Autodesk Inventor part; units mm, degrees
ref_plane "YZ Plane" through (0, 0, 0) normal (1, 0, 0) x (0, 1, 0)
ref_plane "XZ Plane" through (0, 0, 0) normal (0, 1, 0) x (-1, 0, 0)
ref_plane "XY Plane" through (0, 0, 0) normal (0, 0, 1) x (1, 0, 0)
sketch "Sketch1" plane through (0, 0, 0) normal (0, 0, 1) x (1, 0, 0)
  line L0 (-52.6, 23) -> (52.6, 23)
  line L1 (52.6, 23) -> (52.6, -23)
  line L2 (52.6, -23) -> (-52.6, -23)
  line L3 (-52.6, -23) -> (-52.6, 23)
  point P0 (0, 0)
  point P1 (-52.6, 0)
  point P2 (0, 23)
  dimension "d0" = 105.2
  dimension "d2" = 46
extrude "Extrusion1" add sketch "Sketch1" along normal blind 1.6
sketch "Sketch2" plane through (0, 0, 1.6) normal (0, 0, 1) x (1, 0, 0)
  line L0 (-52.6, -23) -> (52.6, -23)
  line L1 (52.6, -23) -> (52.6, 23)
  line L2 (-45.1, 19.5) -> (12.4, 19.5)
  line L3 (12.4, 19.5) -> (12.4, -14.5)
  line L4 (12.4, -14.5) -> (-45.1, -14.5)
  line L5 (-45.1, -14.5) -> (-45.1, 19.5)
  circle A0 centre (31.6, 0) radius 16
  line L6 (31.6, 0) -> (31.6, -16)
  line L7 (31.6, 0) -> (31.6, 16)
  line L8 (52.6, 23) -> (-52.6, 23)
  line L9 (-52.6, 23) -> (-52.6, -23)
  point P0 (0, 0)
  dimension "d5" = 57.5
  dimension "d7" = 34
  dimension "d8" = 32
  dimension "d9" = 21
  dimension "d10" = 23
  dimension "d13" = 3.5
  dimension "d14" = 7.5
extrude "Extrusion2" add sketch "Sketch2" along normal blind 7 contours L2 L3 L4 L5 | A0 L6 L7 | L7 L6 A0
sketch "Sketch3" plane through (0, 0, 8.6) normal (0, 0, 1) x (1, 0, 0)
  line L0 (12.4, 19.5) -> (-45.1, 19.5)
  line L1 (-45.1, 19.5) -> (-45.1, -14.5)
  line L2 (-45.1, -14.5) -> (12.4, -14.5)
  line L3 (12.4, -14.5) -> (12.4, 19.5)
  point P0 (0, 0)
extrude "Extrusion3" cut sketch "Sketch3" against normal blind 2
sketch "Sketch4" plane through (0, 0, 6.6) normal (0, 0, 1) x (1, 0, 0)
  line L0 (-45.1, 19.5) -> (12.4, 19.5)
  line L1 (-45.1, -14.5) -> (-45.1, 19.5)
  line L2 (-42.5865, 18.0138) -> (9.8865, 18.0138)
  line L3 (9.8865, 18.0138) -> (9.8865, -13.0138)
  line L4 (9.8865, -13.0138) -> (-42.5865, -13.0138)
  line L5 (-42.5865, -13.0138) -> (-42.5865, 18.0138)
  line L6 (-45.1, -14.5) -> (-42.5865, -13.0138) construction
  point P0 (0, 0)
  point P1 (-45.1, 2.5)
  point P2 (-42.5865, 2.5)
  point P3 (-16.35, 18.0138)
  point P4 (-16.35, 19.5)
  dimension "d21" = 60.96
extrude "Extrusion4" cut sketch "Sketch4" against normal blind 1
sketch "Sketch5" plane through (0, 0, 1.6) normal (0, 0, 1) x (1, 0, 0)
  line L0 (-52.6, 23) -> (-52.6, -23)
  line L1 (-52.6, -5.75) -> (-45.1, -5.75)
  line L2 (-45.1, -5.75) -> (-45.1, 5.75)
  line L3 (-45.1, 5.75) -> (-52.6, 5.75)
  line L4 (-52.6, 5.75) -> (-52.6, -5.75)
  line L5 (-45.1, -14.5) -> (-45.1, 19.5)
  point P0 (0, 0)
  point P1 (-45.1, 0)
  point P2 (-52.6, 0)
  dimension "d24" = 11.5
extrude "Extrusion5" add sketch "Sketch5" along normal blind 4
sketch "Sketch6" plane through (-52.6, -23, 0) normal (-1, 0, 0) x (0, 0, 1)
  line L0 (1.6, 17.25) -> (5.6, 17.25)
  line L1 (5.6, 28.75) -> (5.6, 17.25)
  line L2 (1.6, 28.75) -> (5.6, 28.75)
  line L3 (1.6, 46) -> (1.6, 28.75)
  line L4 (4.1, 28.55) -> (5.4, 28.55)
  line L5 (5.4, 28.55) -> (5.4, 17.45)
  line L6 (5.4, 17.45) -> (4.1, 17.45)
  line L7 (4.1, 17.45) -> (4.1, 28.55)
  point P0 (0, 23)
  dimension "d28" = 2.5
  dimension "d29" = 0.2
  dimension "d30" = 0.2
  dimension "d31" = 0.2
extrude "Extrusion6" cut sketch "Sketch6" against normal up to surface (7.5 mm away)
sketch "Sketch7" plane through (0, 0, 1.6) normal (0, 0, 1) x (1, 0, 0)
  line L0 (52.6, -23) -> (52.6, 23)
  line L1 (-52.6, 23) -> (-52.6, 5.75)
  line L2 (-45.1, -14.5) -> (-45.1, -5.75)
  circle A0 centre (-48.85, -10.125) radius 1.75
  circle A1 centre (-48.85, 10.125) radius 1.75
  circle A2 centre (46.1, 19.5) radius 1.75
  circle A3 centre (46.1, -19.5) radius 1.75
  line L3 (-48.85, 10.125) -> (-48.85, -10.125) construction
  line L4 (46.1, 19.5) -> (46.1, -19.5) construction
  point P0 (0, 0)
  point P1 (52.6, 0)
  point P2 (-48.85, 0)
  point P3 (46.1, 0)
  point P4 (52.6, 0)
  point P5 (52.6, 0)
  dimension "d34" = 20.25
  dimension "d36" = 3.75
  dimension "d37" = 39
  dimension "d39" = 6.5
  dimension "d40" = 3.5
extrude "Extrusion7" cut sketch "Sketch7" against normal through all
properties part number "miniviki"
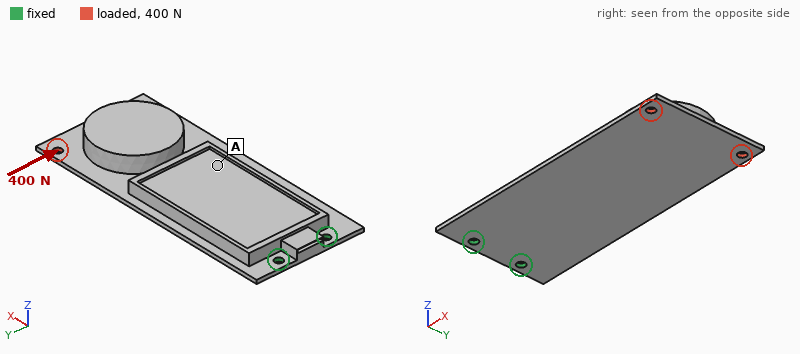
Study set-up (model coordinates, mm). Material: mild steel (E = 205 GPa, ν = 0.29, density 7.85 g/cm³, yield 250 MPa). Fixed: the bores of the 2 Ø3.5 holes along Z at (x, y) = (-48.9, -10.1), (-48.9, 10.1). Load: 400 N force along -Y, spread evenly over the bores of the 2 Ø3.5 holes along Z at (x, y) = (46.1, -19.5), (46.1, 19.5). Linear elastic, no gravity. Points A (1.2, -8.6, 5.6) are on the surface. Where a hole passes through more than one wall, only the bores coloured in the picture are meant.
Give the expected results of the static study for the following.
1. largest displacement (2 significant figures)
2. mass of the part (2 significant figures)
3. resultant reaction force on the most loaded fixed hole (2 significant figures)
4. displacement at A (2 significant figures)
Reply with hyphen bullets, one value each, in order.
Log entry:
- 74 µm
- 170 g
- 1.7 kN
- 26 µm
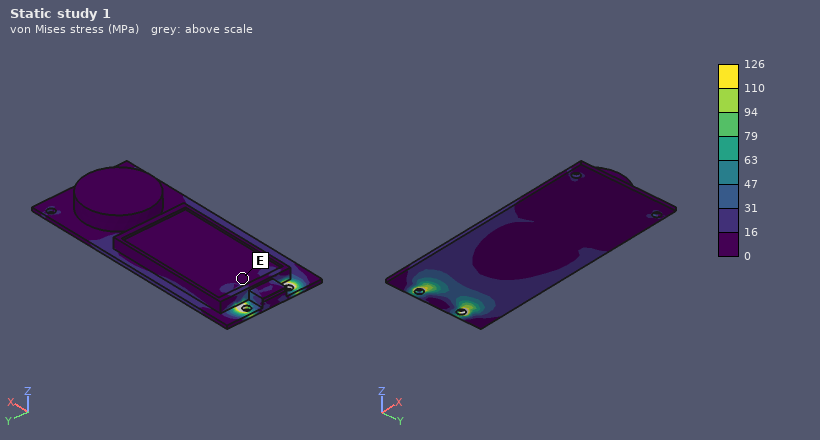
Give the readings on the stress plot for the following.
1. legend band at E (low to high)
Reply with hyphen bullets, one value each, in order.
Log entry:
- 0 to 16 MPa
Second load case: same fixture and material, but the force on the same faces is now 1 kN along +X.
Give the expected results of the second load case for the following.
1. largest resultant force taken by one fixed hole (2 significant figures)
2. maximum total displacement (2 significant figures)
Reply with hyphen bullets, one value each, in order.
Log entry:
- 500 N
- 69 µm
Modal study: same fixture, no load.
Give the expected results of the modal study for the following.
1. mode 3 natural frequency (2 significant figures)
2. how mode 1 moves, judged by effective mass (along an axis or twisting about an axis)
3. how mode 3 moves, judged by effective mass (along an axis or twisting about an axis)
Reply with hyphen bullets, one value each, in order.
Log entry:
- 1700 Hz
- along Z
- along Y
